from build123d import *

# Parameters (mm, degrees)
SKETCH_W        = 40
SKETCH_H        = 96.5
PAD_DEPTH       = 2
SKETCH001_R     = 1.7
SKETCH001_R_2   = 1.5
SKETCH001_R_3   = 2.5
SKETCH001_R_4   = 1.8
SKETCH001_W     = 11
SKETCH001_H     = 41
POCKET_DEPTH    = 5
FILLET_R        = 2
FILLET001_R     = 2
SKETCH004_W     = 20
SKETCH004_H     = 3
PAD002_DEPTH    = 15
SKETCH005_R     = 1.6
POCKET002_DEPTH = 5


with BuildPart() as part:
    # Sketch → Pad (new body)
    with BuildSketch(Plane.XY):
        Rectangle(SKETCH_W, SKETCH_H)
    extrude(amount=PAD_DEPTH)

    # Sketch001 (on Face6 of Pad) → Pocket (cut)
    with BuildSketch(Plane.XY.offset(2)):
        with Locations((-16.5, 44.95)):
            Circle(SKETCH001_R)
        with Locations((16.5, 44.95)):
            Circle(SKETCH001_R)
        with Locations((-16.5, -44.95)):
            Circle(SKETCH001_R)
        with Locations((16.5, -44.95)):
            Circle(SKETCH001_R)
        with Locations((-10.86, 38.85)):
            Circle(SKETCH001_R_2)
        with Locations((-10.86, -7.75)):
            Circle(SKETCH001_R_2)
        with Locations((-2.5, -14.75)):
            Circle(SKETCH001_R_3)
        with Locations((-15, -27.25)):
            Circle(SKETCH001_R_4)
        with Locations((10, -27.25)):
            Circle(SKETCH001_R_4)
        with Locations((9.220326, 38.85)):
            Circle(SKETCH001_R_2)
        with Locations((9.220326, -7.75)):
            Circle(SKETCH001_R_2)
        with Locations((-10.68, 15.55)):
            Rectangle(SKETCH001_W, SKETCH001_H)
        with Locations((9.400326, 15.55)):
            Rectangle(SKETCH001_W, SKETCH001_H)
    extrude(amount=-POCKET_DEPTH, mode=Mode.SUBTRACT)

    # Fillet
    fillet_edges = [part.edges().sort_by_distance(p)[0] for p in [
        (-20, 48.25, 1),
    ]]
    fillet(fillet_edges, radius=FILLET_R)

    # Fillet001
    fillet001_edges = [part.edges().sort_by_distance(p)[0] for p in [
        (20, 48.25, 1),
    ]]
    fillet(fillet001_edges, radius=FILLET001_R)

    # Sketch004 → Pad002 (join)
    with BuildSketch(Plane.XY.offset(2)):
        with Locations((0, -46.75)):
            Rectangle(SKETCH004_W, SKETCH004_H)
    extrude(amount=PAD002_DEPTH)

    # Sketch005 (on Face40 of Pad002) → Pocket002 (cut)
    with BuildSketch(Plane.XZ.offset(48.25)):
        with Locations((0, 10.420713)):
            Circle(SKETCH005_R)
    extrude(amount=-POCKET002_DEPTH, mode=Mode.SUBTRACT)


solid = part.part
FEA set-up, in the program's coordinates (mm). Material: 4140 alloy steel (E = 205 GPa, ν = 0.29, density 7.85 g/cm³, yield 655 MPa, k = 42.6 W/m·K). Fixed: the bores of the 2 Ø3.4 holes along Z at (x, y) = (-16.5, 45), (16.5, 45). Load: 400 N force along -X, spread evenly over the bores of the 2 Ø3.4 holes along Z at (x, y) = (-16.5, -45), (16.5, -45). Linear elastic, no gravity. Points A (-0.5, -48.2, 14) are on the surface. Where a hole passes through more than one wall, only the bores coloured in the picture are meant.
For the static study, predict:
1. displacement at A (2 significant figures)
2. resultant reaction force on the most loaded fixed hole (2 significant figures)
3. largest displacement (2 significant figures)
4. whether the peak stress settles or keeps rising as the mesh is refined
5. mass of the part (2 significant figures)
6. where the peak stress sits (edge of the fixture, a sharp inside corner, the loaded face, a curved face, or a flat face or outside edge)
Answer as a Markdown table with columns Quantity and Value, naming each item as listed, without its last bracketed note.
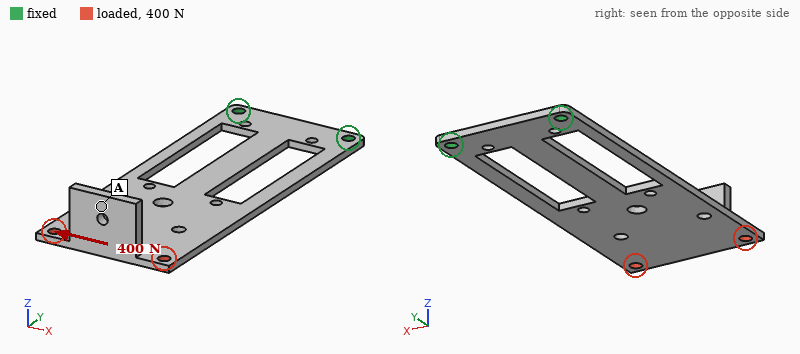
| Quantity | Value |
|---|---|
| displacement at A | 0.20 mm |
| resultant reaction force on the most loaded fixed hole | 1.1 kN |
| largest displacement | 0.20 mm |
| whether the peak stress settles or keeps rising as the mesh is refined | keeps rising |
| mass of the part | 52 g |
| where the peak stress sits | a sharp inside corner |
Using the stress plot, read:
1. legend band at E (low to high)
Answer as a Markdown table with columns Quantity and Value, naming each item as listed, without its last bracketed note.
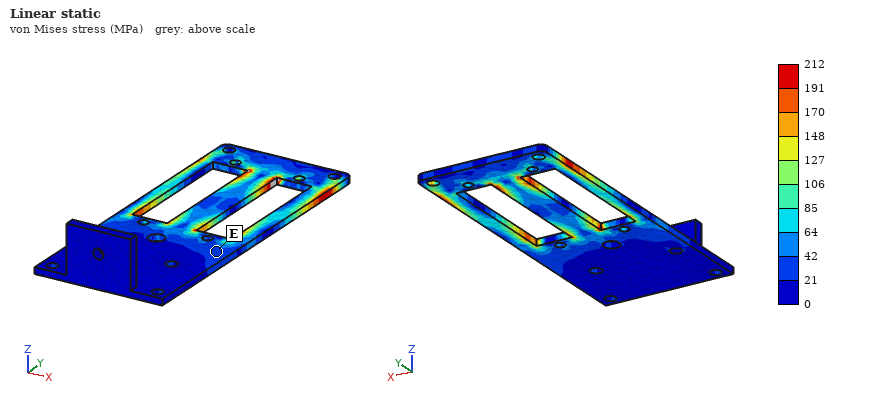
| Quantity | Value |
|---|---|
| legend band at E | 21 to 42 MPa |
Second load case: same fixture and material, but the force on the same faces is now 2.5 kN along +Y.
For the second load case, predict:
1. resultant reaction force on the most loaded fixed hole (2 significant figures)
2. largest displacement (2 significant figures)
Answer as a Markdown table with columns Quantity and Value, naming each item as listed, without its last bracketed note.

| Quantity | Value |
|---|---|
| resultant reaction force on the most loaded fixed hole | 1.3 kN |
| largest displacement | 36 µm |
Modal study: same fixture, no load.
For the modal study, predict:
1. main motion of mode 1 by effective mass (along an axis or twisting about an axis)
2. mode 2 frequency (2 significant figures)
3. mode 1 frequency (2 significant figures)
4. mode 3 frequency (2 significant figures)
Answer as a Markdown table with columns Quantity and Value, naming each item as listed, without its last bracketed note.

| Quantity | Value |
|---|---|
| main motion of mode 1 by effective mass | along Z |
| mode 2 frequency | 630 Hz |
| mode 1 frequency | 110 Hz |
| mode 3 frequency | 930 Hz |
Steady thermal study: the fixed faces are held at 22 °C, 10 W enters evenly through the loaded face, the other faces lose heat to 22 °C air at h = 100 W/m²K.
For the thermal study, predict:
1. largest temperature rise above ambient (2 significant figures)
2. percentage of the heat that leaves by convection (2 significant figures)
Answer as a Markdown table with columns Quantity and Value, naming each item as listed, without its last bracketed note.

| Quantity | Value |
|---|---|
| largest temperature rise above ambient | 72 K |
| percentage of the heat that leaves by convection | 99 % |
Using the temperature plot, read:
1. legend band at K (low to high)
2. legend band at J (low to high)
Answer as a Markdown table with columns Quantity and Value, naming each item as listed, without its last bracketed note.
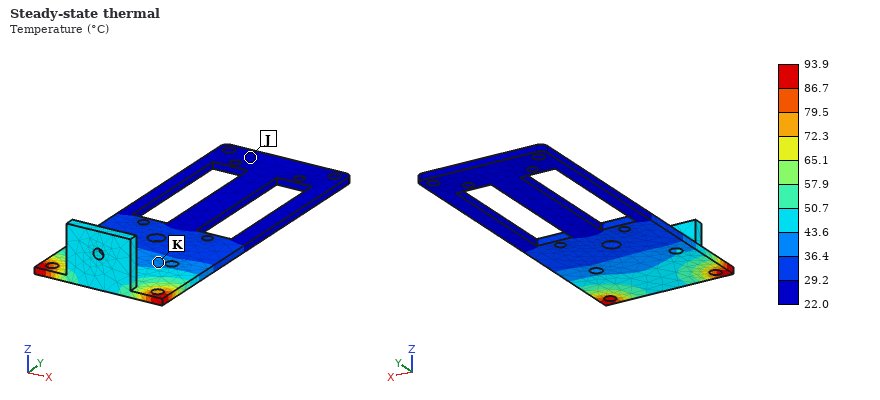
| Quantity | Value |
|---|---|
| legend band at K | 36.4 to 43.6 °C |
| legend band at J | 22.0 to 29.2 °C |
